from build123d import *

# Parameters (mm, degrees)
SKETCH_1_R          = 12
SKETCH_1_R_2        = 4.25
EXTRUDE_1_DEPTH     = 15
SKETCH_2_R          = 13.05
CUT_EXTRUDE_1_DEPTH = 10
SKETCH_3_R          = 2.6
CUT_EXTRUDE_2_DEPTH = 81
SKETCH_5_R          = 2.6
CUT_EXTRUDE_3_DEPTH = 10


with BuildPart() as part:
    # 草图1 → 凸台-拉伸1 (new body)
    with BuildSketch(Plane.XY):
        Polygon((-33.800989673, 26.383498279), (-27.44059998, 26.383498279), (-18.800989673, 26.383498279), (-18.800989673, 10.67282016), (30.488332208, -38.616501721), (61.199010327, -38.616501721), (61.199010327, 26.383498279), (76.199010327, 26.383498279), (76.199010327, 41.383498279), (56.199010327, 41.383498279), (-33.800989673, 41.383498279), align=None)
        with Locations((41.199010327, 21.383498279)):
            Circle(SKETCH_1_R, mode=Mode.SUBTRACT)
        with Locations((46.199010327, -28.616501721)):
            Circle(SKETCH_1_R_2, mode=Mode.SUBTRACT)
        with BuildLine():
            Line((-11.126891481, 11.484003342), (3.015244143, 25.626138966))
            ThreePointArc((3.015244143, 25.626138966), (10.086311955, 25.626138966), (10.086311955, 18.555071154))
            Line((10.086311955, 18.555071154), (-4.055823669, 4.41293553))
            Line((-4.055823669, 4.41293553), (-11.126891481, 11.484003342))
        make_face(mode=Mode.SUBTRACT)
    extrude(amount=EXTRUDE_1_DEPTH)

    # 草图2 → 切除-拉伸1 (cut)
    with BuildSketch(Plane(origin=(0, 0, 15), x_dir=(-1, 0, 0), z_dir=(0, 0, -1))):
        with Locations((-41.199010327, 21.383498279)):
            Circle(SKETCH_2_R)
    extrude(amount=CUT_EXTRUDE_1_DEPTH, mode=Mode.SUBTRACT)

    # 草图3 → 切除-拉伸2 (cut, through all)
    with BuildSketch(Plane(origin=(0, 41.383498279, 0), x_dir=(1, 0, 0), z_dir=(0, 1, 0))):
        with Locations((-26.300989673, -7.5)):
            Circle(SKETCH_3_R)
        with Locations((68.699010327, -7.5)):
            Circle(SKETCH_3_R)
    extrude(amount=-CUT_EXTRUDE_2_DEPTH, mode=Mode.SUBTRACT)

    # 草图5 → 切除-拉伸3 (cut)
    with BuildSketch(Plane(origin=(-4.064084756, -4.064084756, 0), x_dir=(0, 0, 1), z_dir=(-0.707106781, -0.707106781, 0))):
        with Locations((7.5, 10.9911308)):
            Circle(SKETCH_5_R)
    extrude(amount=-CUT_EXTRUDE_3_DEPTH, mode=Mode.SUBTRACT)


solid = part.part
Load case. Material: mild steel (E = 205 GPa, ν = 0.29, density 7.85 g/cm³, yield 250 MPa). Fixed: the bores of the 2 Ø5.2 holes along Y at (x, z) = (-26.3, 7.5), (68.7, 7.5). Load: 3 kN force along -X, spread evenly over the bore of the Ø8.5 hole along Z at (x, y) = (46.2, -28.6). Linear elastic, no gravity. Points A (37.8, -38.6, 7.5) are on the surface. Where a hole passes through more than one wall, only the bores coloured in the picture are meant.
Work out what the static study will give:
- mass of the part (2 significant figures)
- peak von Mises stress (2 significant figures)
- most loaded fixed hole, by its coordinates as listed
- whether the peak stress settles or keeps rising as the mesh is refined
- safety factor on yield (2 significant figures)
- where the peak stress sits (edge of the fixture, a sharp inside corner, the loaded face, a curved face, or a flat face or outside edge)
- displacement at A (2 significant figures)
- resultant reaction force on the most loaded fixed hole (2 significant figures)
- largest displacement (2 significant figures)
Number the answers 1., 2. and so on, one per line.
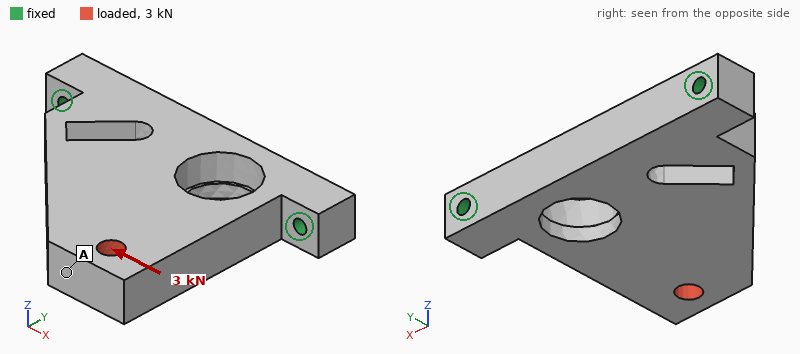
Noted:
1. 560 g
2. 90 MPa
3. (-26.3, 7.5)
4. settles
5. 2.8
6. a curved face
7. 14 µm
8. 3.0 kN
9. 15 µm
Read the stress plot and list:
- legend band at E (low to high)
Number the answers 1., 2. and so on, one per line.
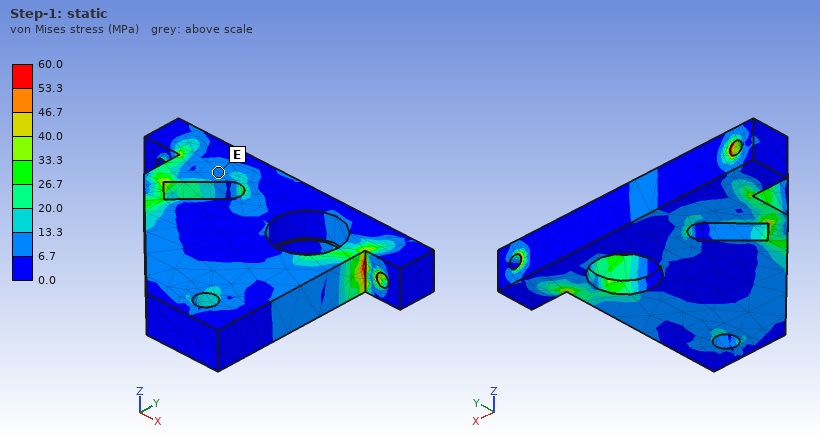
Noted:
1. 6.7 to 13.3 MPa
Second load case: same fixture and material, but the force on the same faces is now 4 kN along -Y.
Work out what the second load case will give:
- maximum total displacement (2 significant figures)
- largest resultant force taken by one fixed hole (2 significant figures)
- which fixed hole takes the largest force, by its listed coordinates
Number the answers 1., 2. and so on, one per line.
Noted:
1. 8.3 µm
2. 3.2 kN
3. (68.7, 7.5)
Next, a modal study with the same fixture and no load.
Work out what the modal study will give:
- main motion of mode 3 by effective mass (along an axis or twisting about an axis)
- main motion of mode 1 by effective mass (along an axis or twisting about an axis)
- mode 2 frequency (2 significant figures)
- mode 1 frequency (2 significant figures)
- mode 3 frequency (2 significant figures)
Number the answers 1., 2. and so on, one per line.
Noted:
1. along X
2. along Z
3. 5000 Hz
4. 1300 Hz
5. 5700 Hz
